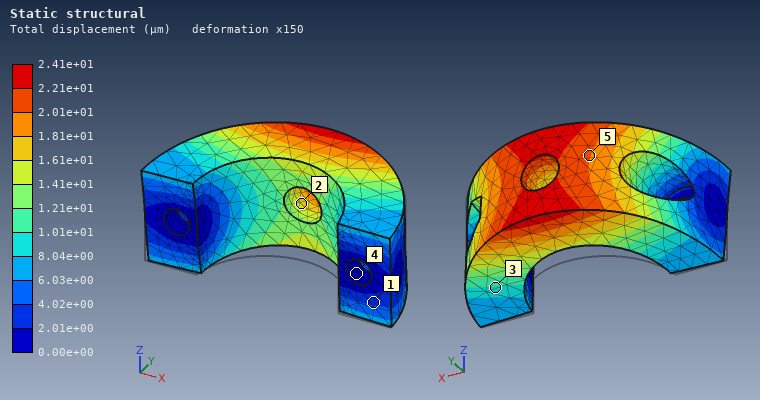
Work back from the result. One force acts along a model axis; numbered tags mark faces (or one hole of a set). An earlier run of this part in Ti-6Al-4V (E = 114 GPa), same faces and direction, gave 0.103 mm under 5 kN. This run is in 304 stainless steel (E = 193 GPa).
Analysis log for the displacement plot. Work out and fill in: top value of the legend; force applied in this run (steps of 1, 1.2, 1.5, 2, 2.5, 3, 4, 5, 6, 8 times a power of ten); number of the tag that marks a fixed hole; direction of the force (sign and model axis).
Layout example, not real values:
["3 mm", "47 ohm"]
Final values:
["2.41e+01 µm", "2 kN", "4", "+Z"]
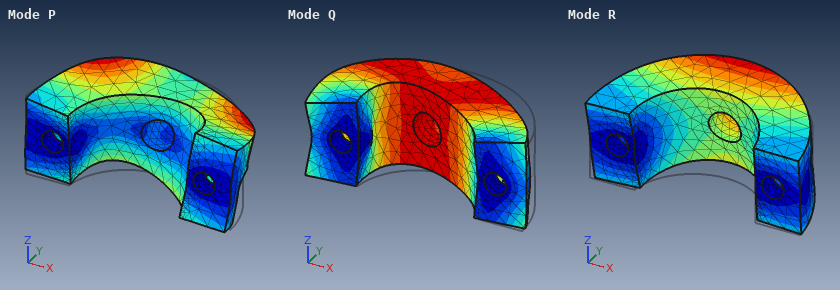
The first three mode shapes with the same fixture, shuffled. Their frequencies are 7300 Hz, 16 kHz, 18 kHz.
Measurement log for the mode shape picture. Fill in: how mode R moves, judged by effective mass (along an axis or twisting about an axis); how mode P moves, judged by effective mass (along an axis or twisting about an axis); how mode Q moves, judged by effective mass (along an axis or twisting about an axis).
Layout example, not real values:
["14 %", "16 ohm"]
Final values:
["along Z", "twisting about Y", "along X"]
